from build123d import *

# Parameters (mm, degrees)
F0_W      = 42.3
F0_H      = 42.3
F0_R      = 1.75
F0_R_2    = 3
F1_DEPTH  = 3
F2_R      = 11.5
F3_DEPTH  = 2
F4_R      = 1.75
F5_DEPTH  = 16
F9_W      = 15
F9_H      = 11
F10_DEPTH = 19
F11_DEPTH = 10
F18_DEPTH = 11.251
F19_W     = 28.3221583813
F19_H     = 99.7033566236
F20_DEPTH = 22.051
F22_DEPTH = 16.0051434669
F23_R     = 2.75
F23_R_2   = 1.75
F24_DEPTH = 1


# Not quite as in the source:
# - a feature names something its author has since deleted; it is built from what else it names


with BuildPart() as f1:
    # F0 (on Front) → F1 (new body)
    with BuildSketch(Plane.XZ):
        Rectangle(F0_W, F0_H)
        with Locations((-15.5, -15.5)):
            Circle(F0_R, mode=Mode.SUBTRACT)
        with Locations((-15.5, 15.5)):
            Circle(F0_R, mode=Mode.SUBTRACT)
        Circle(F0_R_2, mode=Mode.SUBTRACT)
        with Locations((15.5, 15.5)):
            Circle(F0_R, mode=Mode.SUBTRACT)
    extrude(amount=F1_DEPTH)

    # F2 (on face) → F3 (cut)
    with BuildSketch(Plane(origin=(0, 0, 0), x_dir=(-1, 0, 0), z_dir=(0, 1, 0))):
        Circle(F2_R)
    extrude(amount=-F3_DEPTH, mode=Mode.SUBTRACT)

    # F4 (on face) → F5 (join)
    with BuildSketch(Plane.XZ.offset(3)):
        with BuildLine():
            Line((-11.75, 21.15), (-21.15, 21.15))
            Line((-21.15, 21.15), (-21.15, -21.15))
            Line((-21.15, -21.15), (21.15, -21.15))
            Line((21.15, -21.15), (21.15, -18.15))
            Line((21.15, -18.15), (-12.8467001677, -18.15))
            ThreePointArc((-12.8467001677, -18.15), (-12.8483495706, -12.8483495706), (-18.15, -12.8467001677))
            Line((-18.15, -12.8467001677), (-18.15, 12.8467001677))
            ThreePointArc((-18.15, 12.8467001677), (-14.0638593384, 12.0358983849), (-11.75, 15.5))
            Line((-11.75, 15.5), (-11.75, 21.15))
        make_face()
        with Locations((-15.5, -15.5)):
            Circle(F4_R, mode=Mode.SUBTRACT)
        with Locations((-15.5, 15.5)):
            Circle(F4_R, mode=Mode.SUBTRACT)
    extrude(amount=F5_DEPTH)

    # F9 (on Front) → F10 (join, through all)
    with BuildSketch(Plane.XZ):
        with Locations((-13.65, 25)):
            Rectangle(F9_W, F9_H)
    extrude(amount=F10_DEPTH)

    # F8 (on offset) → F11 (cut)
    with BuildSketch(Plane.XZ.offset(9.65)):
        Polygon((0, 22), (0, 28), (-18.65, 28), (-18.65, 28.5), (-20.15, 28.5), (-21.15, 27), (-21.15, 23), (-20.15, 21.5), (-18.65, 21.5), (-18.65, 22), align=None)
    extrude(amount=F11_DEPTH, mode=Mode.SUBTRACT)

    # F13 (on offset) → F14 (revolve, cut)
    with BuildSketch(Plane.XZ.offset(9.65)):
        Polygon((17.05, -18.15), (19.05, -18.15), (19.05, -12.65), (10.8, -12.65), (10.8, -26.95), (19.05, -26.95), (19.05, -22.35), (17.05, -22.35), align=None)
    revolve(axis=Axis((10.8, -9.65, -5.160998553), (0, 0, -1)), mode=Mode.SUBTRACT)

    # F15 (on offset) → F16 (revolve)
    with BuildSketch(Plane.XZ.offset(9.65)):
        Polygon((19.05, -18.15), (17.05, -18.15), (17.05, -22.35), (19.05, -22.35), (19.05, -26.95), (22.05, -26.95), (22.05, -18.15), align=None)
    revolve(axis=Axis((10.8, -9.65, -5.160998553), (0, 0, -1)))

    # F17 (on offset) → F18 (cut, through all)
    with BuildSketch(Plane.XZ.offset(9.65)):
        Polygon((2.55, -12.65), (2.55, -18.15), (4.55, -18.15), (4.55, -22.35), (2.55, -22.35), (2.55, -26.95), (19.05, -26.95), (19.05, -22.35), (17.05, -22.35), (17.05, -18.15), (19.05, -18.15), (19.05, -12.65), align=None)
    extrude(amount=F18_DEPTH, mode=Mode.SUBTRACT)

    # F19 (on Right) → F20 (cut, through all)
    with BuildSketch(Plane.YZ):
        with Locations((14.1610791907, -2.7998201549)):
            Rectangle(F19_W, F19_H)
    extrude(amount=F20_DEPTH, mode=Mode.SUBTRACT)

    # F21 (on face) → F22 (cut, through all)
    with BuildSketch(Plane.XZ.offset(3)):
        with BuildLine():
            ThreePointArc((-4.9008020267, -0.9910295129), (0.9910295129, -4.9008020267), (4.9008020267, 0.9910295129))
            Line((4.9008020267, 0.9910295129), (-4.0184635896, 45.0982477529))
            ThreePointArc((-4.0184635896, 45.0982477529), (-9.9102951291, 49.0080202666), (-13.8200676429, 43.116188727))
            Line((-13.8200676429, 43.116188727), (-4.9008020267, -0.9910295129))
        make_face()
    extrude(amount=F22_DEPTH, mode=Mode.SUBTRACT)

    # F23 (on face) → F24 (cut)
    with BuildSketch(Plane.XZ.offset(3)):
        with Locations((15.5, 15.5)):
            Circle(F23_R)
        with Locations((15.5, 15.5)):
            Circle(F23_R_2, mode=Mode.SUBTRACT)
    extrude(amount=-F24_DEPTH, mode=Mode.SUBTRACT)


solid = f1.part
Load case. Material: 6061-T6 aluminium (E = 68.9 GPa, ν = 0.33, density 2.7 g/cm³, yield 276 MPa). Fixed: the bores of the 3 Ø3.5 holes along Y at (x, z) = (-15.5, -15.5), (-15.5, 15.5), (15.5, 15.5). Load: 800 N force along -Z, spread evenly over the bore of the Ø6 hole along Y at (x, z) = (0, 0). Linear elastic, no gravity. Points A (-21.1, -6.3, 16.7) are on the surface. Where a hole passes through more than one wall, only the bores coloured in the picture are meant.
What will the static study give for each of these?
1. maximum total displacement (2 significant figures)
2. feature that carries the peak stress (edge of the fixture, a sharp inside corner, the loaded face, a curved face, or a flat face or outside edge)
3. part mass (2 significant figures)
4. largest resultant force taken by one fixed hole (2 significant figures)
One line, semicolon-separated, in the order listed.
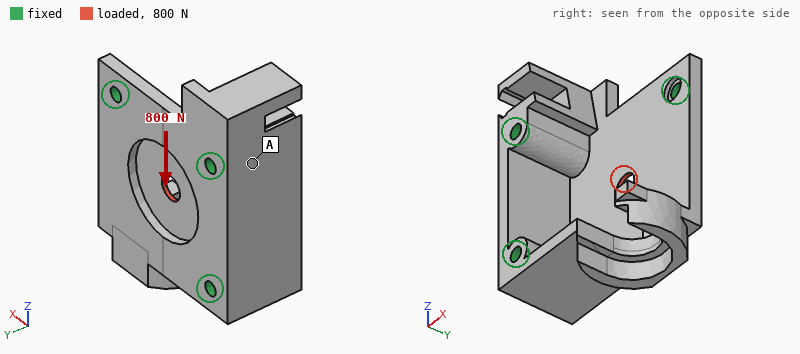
8.0 µm; the loaded face; 30 g; 320 N
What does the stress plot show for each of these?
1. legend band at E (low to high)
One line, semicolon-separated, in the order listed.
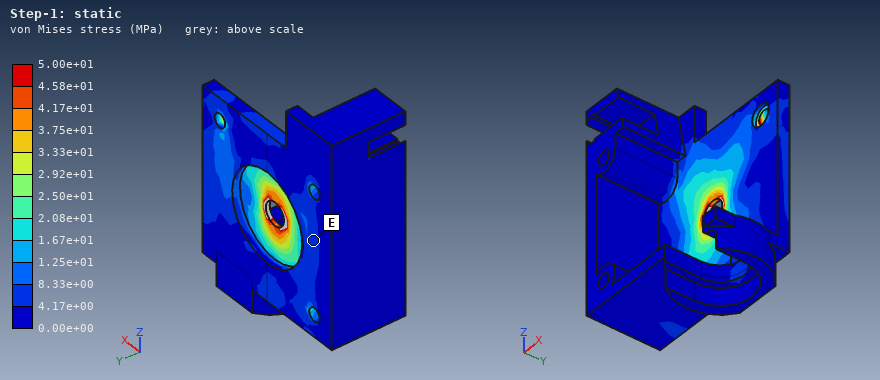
4.17e+00 to 8.33e+00 MPa
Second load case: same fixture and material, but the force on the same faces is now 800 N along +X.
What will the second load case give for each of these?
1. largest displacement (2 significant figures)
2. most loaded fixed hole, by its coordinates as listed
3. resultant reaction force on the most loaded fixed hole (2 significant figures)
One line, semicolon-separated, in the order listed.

7.7 µm; (-15.5, -15.5); 360 N
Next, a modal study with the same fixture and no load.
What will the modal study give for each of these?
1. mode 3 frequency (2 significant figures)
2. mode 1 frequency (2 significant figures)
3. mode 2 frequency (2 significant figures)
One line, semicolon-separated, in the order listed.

9800 Hz; 4400 Hz; 6200 Hz
